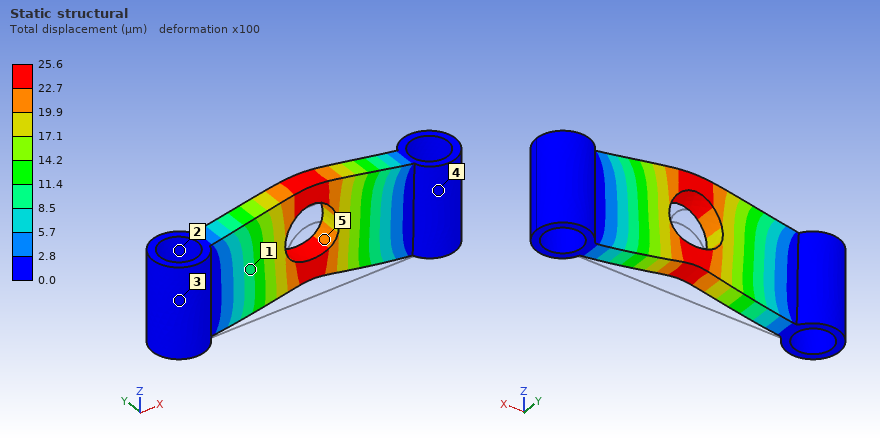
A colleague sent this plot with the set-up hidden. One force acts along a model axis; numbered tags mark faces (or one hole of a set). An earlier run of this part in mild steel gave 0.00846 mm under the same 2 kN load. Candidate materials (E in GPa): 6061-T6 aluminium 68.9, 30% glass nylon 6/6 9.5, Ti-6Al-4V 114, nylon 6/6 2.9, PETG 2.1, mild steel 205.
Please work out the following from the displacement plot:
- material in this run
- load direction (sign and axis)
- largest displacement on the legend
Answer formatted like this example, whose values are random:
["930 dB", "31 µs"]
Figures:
["6061-T6 aluminium", "+Z", "25.6 µm"]
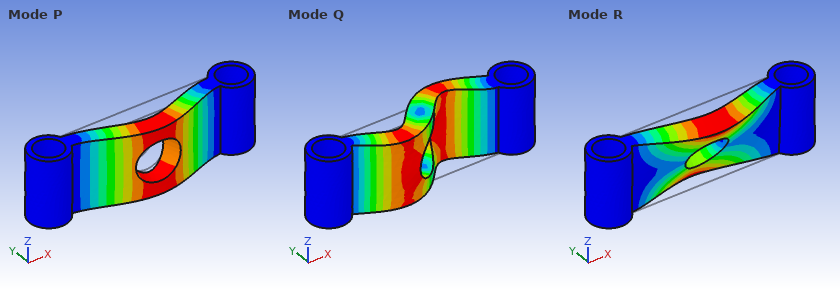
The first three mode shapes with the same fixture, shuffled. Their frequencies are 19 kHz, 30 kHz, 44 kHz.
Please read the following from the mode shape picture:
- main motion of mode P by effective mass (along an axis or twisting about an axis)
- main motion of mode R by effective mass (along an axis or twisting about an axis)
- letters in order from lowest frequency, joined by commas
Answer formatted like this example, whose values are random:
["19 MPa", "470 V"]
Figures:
["along Y", "twisting about X", "P, R, Q"]
